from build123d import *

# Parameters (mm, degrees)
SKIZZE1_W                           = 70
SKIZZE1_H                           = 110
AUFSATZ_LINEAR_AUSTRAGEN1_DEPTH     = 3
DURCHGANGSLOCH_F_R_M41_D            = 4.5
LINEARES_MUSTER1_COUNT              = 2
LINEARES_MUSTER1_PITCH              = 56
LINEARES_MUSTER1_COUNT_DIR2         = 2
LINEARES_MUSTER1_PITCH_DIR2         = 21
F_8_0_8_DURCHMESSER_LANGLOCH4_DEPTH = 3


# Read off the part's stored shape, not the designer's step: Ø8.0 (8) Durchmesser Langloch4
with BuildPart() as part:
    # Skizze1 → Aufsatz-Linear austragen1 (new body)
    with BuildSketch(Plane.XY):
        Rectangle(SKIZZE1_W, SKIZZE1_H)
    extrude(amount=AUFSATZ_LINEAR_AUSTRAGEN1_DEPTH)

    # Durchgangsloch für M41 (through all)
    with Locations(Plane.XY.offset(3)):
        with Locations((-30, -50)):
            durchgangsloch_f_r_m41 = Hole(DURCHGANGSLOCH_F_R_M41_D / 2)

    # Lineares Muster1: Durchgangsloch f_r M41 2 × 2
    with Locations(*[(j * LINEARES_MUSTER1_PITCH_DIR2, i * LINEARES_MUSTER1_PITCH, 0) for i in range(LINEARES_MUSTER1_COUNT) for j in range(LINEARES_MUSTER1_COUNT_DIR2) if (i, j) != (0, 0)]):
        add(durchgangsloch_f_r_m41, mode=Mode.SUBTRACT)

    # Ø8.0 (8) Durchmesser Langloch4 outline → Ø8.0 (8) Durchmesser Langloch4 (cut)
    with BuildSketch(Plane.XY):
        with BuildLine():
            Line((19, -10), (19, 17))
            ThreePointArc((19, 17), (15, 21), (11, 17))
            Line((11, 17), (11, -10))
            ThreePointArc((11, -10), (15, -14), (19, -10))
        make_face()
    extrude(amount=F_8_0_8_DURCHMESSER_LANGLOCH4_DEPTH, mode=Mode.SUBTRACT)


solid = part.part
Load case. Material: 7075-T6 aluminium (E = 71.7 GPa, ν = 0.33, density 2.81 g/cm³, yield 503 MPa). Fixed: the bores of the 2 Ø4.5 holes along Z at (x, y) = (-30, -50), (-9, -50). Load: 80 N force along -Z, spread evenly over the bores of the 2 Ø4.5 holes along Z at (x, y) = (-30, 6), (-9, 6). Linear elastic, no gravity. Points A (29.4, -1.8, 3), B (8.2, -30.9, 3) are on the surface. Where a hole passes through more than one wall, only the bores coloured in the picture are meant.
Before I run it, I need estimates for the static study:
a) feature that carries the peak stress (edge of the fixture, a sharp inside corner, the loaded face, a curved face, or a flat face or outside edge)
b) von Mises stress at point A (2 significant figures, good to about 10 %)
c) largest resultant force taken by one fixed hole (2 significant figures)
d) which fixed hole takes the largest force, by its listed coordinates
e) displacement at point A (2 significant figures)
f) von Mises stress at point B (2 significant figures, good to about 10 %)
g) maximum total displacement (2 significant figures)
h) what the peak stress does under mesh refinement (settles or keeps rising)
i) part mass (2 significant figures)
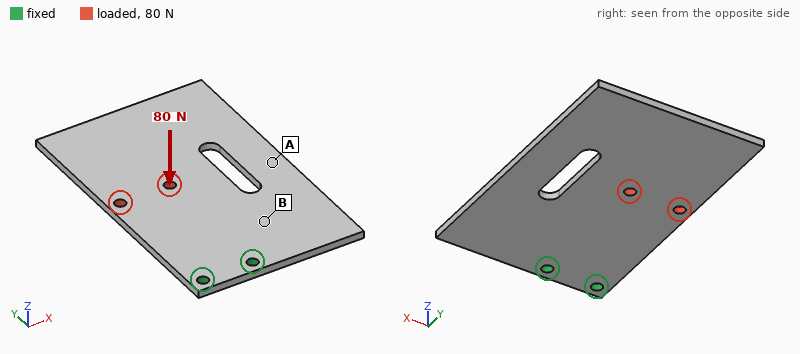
edge of the fixture
11 MPa
55 N
(-9, -50)
0.37 mm
23 MPa
1.3 mm
keeps rising
62 g
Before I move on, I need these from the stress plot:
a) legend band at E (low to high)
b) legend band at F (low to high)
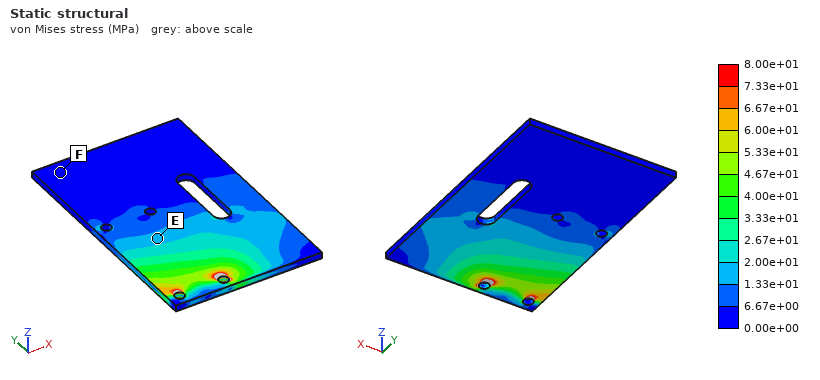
1.33e+01 to 2.00e+01 MPa
0.00e+00 to 6.67e+00 MPa
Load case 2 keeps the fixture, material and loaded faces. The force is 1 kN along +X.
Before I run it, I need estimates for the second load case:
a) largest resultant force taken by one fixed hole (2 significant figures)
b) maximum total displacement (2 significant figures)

2.4 kN
0.18 mm
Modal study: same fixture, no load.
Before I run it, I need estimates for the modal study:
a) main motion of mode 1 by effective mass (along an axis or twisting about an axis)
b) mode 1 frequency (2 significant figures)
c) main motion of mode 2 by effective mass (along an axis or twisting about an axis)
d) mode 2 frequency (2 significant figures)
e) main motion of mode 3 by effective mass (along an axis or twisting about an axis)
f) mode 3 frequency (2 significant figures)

along Z
200 Hz
twisting about Y
580 Hz
along Z
1200 Hz
